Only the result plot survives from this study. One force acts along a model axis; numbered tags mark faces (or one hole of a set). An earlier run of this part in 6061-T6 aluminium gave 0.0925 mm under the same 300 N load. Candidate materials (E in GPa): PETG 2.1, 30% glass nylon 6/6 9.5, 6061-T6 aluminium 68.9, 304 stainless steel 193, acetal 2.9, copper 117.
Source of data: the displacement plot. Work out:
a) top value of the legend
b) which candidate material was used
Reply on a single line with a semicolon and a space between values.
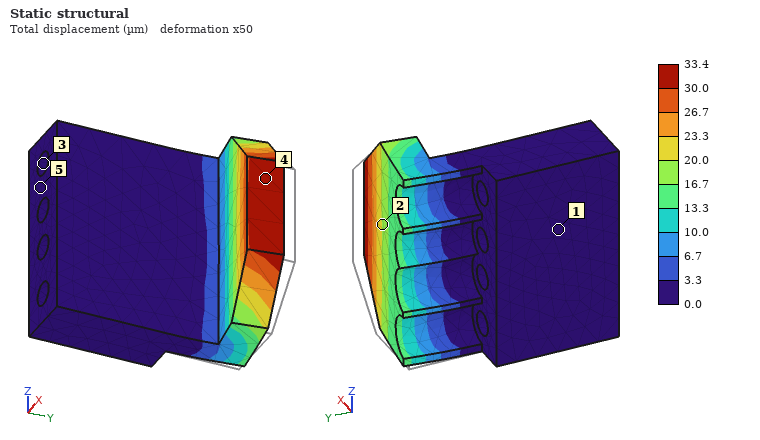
33.4 µm; 304 stainless steel
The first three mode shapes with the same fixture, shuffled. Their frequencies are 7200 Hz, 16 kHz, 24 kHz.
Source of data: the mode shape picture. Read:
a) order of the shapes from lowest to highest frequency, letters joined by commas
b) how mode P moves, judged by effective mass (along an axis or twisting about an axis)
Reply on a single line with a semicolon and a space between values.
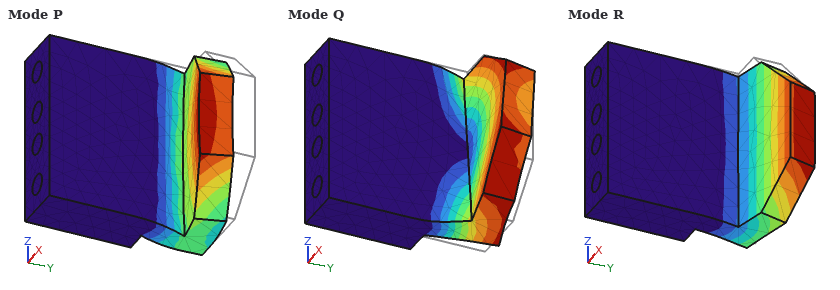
R, Q, P; along X
